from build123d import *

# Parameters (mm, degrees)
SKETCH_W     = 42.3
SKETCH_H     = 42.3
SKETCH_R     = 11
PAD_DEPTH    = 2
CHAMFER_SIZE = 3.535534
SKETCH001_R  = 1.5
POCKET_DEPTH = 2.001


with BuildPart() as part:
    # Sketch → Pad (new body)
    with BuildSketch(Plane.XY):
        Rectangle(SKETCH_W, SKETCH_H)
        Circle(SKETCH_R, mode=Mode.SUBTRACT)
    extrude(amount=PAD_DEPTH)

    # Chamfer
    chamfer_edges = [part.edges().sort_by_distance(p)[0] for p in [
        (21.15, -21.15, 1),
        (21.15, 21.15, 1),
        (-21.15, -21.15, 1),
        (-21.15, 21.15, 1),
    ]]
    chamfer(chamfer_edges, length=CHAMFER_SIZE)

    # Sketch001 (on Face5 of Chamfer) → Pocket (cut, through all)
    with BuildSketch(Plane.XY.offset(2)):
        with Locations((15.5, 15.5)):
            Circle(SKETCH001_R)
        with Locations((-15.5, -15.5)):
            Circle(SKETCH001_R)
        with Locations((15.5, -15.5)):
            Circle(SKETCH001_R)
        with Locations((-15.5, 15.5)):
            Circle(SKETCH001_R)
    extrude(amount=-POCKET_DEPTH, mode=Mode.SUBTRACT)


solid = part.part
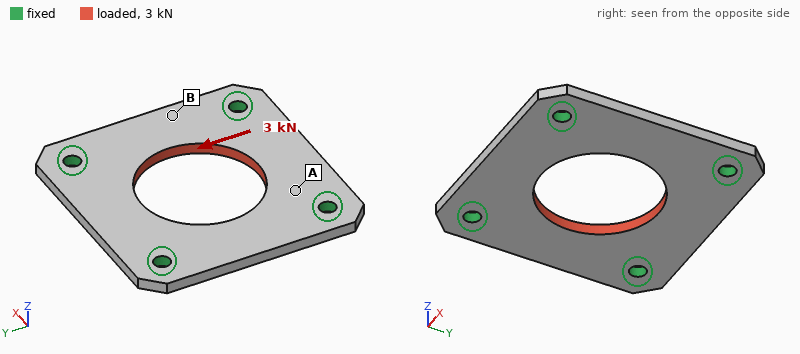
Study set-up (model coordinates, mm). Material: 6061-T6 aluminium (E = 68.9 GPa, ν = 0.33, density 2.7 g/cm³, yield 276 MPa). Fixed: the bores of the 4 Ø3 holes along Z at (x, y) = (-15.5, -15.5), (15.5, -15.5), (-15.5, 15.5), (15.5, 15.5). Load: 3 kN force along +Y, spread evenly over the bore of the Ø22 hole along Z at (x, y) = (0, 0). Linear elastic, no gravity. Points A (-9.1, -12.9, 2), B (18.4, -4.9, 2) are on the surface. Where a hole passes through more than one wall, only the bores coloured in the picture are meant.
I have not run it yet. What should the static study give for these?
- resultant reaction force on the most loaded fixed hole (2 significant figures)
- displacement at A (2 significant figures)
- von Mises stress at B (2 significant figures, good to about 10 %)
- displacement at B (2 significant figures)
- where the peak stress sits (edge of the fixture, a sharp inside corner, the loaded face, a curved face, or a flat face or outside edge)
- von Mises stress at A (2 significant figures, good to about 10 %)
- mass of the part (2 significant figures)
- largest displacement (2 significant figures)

770 N
6.9 µm
17 MPa
3.1 µm
edge of the fixture
31 MPa
7.3 g
14 µm
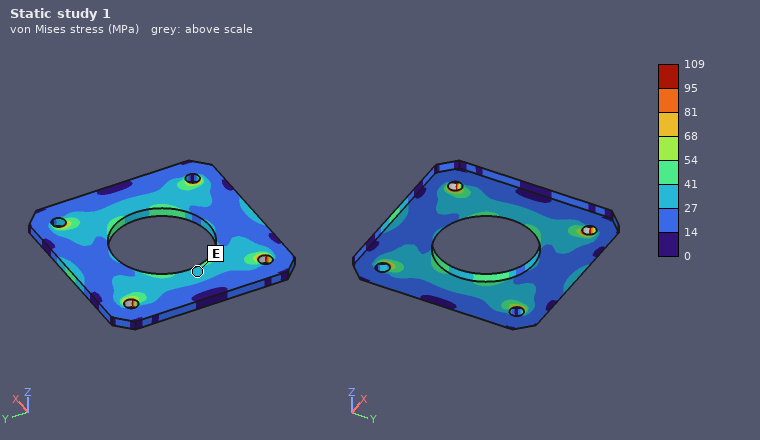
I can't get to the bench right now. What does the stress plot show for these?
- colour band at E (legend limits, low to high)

27 to 41 MPa
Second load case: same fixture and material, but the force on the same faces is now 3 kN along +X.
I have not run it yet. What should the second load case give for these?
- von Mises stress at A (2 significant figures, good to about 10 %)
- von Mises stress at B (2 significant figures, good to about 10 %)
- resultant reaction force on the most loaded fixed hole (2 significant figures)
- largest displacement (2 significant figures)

33 MPa
21 MPa
770 N
14 µm
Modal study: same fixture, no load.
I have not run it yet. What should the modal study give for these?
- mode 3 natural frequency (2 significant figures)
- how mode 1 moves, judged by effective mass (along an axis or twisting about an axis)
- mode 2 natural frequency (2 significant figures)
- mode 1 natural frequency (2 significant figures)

12 kHz
along Z
12 kHz
11 kHz
